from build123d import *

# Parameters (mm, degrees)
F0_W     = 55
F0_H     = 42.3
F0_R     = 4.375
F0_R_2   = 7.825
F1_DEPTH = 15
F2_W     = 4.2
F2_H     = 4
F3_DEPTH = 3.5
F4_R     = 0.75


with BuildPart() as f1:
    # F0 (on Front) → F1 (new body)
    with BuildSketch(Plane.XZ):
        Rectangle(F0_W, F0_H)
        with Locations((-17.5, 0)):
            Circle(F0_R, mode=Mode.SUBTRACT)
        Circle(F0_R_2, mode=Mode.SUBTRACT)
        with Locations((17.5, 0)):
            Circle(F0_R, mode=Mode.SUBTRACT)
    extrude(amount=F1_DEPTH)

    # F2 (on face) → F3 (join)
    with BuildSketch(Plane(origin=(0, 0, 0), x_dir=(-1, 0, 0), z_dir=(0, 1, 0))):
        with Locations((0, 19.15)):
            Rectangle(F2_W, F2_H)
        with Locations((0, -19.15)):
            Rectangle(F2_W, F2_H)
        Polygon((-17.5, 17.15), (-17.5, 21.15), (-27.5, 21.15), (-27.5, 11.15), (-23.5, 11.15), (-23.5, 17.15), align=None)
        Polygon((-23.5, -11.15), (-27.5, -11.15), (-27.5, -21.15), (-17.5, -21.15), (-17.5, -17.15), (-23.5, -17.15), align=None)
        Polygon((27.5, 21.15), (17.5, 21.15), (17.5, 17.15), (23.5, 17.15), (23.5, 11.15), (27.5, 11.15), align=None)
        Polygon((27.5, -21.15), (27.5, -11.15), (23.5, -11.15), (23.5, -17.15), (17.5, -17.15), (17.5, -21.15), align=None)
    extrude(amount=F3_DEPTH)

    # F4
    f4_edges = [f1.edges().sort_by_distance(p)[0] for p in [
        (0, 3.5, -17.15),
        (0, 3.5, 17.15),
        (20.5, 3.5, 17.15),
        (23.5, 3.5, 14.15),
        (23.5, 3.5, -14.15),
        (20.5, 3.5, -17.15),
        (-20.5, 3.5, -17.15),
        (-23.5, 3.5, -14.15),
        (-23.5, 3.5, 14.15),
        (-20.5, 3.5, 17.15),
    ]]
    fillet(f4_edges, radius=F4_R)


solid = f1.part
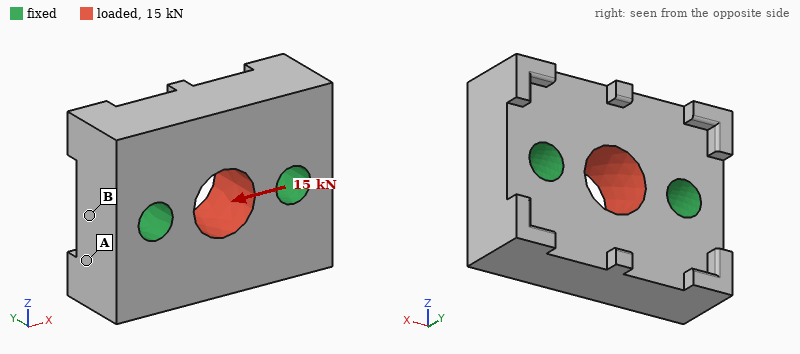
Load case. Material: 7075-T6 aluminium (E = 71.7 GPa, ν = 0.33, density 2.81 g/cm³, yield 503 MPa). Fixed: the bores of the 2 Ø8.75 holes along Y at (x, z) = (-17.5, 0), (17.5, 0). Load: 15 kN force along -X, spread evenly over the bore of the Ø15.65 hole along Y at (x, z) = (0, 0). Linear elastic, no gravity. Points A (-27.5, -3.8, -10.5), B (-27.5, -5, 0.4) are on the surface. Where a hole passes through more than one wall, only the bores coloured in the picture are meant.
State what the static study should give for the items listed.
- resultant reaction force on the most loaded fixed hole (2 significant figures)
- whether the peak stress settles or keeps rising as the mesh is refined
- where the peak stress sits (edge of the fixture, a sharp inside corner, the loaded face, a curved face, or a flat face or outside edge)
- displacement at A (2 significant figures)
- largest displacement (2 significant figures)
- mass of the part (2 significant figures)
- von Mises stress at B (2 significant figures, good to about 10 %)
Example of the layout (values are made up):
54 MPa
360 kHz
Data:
7.5 kN
keeps rising
edge of the fixture
2.1 µm
5.8 µm
88 g
11 MPa
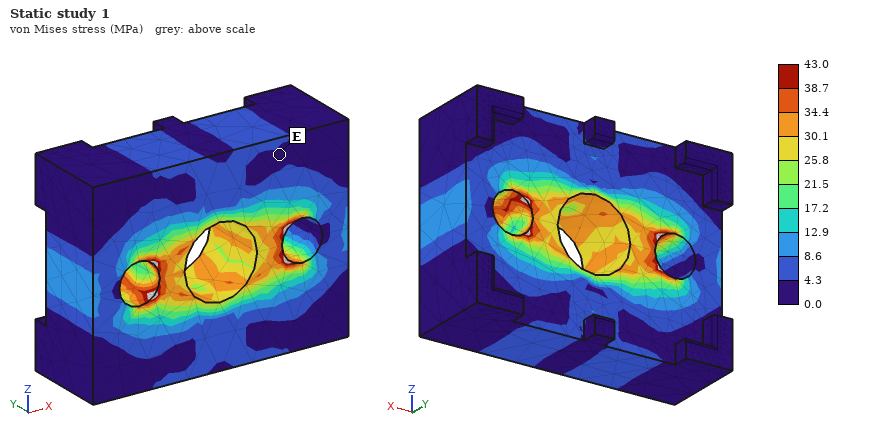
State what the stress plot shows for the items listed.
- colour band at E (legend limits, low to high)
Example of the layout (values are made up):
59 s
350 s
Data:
0.0 to 4.3 MPa
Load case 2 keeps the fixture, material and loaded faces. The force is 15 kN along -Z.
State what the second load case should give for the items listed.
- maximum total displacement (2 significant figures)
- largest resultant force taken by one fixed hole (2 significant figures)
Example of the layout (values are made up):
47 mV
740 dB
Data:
8.5 µm
7.5 kN
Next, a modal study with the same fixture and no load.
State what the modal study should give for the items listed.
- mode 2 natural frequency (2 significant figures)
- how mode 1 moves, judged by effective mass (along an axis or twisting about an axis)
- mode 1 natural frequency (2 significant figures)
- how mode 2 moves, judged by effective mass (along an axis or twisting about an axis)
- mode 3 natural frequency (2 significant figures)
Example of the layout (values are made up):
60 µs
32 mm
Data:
21 kHz
twisting about X
19 kHz
along Y
25 kHz
